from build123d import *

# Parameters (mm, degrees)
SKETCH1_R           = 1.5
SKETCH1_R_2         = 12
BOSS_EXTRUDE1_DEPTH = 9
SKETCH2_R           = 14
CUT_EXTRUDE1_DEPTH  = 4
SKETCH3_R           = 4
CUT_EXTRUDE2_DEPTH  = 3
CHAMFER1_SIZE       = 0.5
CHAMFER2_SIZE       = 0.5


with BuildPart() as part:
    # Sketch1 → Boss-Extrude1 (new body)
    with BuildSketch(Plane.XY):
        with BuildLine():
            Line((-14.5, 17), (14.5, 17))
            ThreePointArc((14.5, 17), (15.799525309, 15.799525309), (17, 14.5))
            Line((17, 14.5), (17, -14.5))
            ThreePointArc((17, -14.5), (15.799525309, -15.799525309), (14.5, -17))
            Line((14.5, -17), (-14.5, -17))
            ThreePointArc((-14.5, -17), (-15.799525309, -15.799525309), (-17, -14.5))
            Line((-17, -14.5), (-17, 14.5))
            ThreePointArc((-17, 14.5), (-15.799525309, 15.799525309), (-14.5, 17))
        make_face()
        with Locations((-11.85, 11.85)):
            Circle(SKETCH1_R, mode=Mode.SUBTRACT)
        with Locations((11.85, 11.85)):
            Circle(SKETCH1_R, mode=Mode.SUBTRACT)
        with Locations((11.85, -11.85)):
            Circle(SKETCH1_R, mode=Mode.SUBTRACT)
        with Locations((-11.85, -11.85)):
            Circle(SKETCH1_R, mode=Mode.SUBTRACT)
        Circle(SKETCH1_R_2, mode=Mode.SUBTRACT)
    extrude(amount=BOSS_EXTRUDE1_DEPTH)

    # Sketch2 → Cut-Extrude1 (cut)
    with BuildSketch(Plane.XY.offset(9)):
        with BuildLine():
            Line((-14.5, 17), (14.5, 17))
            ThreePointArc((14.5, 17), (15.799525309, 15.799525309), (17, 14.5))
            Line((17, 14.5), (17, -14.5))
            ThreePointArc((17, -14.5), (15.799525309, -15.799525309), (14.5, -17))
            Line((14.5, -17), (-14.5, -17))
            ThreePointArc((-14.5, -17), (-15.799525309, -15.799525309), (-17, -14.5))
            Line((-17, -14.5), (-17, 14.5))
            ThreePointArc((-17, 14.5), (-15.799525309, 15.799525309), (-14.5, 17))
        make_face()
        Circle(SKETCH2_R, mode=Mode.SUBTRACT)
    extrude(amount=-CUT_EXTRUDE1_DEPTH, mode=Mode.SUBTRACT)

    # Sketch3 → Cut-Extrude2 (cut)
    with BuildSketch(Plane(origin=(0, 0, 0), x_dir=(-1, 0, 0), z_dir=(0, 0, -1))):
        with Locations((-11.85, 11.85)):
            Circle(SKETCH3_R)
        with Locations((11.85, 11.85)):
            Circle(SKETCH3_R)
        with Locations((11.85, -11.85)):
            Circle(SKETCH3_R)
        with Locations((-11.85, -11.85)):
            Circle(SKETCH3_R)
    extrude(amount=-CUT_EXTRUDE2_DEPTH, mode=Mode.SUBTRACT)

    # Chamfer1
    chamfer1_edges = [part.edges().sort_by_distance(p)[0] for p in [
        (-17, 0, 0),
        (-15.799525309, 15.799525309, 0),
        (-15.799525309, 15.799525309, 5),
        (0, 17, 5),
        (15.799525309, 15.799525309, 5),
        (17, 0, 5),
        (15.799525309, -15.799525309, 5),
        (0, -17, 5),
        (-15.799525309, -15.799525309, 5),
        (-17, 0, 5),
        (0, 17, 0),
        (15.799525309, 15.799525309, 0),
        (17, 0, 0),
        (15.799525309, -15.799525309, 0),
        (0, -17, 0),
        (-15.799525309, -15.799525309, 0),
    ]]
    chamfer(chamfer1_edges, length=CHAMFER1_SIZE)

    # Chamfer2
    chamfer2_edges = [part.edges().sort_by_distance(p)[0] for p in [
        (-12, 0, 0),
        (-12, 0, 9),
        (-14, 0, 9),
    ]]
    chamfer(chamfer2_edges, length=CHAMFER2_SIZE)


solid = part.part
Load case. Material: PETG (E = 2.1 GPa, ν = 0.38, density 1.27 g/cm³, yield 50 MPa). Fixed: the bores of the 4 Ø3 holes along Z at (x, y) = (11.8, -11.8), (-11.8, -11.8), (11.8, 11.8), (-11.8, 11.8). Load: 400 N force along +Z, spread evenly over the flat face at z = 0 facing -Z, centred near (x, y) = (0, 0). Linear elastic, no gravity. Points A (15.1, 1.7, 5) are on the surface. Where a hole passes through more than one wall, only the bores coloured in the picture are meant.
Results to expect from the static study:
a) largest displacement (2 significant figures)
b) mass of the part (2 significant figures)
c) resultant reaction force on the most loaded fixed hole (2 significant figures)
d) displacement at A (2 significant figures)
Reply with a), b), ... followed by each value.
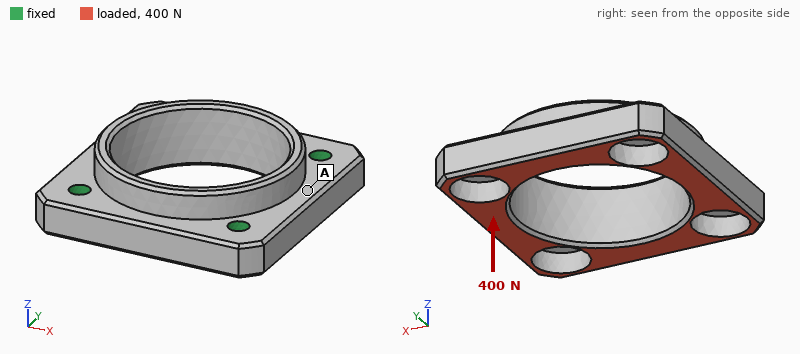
a) 60 µm
b) 4.3 g
c) 100 N
d) 51 µm
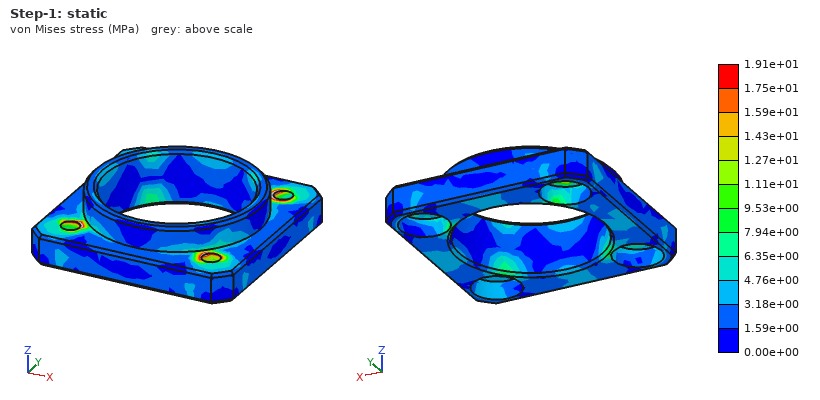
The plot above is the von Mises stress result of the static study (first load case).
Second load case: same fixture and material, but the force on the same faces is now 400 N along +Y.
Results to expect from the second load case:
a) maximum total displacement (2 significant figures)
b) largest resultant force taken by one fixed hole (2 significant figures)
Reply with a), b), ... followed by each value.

a) 96 µm
b) 100 N
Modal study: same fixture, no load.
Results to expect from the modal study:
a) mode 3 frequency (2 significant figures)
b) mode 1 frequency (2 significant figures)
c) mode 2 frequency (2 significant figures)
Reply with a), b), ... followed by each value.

a) 7000 Hz
b) 5700 Hz
c) 7000 Hz
